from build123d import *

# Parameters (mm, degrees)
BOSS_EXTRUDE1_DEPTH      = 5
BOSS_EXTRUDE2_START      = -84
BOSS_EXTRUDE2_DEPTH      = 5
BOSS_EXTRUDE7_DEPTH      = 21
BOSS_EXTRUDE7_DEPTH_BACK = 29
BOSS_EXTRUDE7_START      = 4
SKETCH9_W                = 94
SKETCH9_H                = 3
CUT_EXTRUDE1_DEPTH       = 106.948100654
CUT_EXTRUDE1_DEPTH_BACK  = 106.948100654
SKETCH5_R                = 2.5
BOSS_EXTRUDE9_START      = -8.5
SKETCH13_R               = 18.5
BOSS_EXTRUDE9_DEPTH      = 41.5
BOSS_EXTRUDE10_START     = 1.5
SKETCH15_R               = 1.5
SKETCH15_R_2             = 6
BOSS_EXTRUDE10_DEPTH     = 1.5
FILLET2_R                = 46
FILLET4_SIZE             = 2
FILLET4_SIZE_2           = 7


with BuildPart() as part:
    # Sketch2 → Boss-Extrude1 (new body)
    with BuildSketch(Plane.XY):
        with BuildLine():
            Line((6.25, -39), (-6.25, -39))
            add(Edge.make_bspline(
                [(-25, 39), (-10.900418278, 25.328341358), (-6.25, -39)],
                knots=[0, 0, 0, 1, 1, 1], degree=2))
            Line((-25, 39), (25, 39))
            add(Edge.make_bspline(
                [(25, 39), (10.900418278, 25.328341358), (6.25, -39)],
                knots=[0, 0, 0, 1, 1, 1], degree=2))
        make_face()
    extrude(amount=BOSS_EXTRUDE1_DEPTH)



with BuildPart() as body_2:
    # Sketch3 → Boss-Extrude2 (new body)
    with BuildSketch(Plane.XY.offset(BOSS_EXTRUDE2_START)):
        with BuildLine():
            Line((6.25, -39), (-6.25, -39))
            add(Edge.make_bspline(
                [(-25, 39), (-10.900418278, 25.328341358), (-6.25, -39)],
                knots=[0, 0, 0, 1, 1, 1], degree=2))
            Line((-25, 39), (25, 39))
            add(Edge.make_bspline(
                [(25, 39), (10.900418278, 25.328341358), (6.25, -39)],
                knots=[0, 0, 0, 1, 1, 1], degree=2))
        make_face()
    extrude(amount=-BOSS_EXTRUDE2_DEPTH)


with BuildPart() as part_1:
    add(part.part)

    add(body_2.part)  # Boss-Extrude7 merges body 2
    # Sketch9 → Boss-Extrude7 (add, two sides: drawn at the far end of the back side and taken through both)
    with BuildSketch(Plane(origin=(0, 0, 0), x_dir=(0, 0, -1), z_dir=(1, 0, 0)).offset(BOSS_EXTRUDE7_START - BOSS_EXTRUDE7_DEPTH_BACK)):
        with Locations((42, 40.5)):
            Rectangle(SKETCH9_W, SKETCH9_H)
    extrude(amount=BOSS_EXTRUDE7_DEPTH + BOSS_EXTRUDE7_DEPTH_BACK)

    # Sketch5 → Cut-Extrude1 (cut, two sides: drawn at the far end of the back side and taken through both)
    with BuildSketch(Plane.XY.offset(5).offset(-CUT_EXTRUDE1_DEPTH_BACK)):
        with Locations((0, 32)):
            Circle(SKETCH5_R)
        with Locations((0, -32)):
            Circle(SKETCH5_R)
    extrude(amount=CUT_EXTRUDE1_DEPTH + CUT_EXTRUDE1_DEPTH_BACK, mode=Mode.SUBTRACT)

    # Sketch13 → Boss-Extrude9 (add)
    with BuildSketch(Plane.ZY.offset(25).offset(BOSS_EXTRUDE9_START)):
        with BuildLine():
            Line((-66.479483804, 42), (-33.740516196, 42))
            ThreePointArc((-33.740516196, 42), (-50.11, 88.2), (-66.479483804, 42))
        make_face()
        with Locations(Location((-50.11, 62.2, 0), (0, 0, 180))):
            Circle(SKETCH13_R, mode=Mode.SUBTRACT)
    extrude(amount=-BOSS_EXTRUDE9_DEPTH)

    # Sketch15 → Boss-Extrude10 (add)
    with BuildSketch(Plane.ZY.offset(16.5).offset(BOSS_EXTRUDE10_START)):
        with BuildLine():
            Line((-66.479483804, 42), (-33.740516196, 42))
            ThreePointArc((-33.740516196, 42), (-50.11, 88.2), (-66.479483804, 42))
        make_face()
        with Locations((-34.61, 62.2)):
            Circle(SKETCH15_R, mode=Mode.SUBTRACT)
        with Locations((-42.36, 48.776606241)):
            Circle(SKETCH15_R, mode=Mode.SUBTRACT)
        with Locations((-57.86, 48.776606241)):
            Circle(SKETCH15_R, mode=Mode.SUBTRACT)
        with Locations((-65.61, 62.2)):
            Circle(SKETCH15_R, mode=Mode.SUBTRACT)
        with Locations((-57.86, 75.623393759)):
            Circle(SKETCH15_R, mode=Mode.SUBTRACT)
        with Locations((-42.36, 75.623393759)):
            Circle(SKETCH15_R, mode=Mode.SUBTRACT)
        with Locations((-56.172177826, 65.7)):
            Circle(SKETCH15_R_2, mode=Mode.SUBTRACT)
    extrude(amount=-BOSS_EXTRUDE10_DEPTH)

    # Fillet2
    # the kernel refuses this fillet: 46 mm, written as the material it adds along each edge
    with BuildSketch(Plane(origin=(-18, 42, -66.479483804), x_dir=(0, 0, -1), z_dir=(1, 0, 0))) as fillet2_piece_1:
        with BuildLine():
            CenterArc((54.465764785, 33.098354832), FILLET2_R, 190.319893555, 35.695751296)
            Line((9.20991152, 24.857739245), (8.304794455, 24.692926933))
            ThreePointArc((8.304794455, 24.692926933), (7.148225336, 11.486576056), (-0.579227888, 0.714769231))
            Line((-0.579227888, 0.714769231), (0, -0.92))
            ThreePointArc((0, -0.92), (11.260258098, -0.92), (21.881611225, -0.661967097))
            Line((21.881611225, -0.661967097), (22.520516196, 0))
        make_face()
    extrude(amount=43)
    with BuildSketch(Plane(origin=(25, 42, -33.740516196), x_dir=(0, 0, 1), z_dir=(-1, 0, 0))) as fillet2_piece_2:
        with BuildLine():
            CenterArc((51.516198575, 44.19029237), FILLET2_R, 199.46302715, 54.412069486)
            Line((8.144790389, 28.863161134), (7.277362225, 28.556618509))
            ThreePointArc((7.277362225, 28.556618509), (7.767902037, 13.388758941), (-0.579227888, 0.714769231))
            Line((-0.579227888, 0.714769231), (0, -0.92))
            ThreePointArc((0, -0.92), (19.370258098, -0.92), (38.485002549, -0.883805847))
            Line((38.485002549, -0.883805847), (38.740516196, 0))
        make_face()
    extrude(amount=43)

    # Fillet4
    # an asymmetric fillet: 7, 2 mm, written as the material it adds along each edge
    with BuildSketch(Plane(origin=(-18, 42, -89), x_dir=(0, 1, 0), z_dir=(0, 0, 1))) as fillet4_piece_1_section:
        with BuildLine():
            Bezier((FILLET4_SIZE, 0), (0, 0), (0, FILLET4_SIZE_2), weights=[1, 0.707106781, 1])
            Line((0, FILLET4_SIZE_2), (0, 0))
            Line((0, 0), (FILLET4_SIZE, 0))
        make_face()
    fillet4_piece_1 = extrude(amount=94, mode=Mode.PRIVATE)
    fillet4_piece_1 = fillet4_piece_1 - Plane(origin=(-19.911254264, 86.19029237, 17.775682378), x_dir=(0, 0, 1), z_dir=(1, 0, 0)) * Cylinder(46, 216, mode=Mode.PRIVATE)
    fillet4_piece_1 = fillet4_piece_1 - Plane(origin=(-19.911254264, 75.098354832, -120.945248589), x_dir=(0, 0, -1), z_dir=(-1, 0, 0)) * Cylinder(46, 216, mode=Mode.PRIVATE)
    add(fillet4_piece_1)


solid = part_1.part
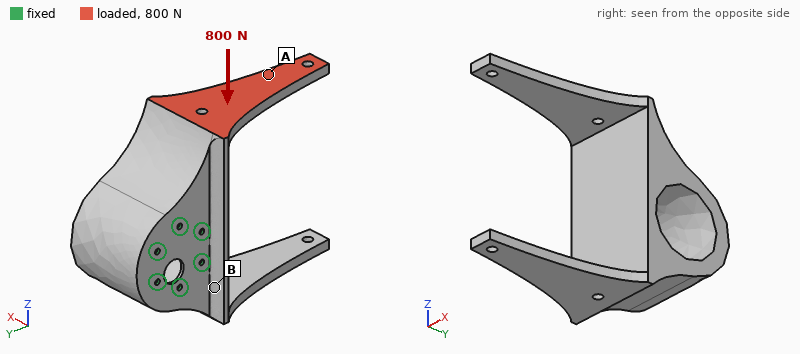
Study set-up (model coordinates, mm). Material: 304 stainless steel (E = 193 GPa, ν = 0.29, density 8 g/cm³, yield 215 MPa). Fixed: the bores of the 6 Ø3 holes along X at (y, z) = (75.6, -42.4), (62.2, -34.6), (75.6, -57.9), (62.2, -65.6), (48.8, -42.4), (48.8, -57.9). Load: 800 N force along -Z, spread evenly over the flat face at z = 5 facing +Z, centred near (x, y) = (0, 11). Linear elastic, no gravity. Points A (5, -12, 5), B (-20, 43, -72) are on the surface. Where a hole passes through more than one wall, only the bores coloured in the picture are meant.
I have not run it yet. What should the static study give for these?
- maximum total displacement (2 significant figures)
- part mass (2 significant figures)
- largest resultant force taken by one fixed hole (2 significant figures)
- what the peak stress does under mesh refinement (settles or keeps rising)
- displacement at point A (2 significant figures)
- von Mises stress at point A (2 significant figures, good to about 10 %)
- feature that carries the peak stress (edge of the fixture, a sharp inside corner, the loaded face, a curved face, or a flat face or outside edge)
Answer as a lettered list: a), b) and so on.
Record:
a) 0.71 mm
b) 760 g
c) 750 N
d) keeps rising
e) 0.41 mm
f) 27 MPa
g) a sharp inside corner
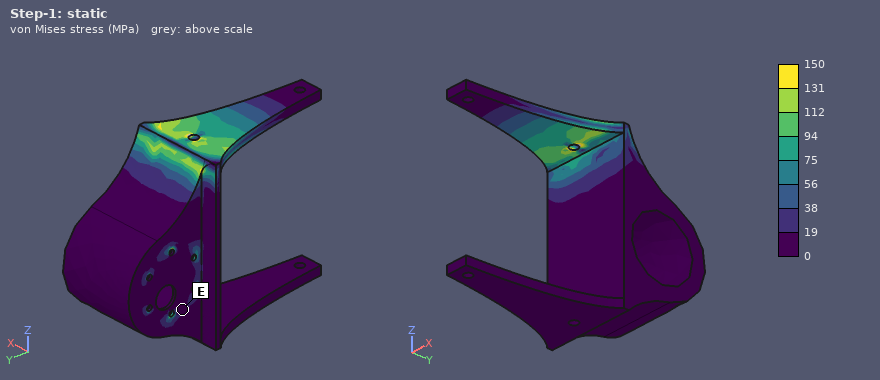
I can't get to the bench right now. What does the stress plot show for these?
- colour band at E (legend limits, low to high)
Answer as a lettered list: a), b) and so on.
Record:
a) 0 to 19 MPa
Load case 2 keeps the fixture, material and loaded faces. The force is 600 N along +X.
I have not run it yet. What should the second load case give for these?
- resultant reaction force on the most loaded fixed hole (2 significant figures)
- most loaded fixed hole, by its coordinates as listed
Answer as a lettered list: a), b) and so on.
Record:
a) 940 N
b) (48.8, -42.4)
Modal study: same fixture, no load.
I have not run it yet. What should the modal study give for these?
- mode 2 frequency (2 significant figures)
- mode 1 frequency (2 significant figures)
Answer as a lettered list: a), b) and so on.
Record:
a) 870 Hz
b) 790 Hz
